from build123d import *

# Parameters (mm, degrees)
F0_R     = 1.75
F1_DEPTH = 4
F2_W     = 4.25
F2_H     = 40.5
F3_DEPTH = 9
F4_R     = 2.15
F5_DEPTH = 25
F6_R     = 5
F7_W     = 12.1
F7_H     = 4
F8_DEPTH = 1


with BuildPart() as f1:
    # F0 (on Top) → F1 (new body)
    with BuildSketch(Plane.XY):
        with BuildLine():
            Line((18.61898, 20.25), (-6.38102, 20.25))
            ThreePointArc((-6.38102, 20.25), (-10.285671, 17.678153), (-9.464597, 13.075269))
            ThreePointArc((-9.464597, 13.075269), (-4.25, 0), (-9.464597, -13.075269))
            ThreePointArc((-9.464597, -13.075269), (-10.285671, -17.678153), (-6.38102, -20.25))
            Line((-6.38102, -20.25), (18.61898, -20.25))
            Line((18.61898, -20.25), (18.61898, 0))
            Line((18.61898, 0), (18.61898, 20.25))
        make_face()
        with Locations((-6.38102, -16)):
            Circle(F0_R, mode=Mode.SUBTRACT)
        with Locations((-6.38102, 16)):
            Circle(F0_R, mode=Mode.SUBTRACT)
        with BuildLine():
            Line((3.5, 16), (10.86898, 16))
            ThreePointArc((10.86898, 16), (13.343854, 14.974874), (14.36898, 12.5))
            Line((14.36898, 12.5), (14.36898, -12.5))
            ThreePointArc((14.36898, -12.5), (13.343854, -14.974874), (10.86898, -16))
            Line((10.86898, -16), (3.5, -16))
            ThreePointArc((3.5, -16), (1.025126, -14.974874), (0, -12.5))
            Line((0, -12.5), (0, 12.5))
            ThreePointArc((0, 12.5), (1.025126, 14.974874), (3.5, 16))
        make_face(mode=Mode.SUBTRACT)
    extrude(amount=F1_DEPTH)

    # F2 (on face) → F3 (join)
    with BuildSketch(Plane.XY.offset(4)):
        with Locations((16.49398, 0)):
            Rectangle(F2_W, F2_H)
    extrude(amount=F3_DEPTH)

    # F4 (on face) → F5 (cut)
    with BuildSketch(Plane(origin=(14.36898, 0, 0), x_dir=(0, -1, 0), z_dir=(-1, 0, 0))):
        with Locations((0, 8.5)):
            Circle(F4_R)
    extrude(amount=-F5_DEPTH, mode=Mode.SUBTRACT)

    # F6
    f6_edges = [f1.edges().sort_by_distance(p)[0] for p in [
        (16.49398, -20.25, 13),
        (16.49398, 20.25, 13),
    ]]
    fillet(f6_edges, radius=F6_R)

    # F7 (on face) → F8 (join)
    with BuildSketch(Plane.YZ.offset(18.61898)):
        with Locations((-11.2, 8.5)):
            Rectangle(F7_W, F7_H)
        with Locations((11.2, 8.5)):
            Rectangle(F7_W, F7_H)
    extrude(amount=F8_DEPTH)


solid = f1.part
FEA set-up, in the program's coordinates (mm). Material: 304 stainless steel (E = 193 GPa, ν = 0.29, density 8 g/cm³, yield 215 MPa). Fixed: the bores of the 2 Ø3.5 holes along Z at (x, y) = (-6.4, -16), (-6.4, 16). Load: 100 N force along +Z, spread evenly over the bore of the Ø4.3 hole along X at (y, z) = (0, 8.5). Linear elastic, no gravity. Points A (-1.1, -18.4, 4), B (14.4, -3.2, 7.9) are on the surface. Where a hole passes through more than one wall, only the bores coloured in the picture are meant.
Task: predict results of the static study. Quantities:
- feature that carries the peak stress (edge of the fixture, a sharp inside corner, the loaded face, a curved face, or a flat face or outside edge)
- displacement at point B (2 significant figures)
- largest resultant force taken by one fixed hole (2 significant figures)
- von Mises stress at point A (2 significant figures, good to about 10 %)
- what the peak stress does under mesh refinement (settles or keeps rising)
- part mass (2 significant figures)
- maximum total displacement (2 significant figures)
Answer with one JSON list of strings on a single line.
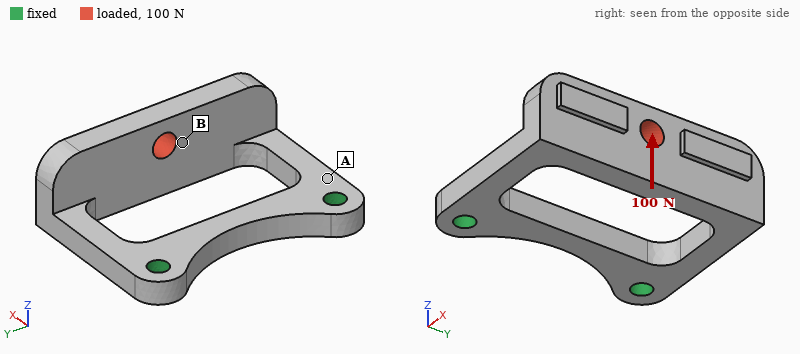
["edge of the fixture", "30 µm", "50 N", "53 MPa", "keeps rising", "31 g", "44 µm"]
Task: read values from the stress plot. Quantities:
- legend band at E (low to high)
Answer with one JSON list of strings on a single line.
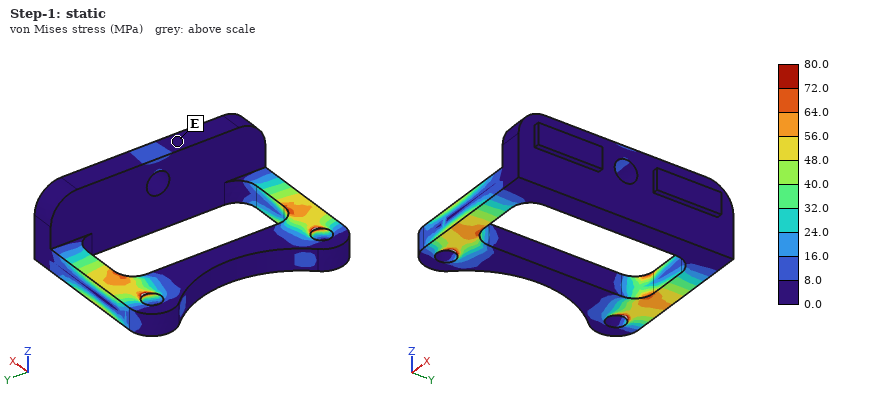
["0.0 to 8.0 MPa"]
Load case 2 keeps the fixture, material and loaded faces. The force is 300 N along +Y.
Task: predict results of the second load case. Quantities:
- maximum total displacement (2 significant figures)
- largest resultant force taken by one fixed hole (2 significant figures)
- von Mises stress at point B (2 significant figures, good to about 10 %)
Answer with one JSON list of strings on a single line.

["26 µm", "200 N", "9.2 MPa"]
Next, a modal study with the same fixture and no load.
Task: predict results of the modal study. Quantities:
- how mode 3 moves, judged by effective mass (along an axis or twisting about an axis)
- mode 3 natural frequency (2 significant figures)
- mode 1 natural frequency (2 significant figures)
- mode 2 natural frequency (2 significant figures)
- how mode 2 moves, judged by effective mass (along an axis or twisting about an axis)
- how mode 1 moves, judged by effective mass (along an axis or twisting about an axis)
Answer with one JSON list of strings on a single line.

["along Y", "5500 Hz", "1900 Hz", "4200 Hz", "along Y", "along Z"]
